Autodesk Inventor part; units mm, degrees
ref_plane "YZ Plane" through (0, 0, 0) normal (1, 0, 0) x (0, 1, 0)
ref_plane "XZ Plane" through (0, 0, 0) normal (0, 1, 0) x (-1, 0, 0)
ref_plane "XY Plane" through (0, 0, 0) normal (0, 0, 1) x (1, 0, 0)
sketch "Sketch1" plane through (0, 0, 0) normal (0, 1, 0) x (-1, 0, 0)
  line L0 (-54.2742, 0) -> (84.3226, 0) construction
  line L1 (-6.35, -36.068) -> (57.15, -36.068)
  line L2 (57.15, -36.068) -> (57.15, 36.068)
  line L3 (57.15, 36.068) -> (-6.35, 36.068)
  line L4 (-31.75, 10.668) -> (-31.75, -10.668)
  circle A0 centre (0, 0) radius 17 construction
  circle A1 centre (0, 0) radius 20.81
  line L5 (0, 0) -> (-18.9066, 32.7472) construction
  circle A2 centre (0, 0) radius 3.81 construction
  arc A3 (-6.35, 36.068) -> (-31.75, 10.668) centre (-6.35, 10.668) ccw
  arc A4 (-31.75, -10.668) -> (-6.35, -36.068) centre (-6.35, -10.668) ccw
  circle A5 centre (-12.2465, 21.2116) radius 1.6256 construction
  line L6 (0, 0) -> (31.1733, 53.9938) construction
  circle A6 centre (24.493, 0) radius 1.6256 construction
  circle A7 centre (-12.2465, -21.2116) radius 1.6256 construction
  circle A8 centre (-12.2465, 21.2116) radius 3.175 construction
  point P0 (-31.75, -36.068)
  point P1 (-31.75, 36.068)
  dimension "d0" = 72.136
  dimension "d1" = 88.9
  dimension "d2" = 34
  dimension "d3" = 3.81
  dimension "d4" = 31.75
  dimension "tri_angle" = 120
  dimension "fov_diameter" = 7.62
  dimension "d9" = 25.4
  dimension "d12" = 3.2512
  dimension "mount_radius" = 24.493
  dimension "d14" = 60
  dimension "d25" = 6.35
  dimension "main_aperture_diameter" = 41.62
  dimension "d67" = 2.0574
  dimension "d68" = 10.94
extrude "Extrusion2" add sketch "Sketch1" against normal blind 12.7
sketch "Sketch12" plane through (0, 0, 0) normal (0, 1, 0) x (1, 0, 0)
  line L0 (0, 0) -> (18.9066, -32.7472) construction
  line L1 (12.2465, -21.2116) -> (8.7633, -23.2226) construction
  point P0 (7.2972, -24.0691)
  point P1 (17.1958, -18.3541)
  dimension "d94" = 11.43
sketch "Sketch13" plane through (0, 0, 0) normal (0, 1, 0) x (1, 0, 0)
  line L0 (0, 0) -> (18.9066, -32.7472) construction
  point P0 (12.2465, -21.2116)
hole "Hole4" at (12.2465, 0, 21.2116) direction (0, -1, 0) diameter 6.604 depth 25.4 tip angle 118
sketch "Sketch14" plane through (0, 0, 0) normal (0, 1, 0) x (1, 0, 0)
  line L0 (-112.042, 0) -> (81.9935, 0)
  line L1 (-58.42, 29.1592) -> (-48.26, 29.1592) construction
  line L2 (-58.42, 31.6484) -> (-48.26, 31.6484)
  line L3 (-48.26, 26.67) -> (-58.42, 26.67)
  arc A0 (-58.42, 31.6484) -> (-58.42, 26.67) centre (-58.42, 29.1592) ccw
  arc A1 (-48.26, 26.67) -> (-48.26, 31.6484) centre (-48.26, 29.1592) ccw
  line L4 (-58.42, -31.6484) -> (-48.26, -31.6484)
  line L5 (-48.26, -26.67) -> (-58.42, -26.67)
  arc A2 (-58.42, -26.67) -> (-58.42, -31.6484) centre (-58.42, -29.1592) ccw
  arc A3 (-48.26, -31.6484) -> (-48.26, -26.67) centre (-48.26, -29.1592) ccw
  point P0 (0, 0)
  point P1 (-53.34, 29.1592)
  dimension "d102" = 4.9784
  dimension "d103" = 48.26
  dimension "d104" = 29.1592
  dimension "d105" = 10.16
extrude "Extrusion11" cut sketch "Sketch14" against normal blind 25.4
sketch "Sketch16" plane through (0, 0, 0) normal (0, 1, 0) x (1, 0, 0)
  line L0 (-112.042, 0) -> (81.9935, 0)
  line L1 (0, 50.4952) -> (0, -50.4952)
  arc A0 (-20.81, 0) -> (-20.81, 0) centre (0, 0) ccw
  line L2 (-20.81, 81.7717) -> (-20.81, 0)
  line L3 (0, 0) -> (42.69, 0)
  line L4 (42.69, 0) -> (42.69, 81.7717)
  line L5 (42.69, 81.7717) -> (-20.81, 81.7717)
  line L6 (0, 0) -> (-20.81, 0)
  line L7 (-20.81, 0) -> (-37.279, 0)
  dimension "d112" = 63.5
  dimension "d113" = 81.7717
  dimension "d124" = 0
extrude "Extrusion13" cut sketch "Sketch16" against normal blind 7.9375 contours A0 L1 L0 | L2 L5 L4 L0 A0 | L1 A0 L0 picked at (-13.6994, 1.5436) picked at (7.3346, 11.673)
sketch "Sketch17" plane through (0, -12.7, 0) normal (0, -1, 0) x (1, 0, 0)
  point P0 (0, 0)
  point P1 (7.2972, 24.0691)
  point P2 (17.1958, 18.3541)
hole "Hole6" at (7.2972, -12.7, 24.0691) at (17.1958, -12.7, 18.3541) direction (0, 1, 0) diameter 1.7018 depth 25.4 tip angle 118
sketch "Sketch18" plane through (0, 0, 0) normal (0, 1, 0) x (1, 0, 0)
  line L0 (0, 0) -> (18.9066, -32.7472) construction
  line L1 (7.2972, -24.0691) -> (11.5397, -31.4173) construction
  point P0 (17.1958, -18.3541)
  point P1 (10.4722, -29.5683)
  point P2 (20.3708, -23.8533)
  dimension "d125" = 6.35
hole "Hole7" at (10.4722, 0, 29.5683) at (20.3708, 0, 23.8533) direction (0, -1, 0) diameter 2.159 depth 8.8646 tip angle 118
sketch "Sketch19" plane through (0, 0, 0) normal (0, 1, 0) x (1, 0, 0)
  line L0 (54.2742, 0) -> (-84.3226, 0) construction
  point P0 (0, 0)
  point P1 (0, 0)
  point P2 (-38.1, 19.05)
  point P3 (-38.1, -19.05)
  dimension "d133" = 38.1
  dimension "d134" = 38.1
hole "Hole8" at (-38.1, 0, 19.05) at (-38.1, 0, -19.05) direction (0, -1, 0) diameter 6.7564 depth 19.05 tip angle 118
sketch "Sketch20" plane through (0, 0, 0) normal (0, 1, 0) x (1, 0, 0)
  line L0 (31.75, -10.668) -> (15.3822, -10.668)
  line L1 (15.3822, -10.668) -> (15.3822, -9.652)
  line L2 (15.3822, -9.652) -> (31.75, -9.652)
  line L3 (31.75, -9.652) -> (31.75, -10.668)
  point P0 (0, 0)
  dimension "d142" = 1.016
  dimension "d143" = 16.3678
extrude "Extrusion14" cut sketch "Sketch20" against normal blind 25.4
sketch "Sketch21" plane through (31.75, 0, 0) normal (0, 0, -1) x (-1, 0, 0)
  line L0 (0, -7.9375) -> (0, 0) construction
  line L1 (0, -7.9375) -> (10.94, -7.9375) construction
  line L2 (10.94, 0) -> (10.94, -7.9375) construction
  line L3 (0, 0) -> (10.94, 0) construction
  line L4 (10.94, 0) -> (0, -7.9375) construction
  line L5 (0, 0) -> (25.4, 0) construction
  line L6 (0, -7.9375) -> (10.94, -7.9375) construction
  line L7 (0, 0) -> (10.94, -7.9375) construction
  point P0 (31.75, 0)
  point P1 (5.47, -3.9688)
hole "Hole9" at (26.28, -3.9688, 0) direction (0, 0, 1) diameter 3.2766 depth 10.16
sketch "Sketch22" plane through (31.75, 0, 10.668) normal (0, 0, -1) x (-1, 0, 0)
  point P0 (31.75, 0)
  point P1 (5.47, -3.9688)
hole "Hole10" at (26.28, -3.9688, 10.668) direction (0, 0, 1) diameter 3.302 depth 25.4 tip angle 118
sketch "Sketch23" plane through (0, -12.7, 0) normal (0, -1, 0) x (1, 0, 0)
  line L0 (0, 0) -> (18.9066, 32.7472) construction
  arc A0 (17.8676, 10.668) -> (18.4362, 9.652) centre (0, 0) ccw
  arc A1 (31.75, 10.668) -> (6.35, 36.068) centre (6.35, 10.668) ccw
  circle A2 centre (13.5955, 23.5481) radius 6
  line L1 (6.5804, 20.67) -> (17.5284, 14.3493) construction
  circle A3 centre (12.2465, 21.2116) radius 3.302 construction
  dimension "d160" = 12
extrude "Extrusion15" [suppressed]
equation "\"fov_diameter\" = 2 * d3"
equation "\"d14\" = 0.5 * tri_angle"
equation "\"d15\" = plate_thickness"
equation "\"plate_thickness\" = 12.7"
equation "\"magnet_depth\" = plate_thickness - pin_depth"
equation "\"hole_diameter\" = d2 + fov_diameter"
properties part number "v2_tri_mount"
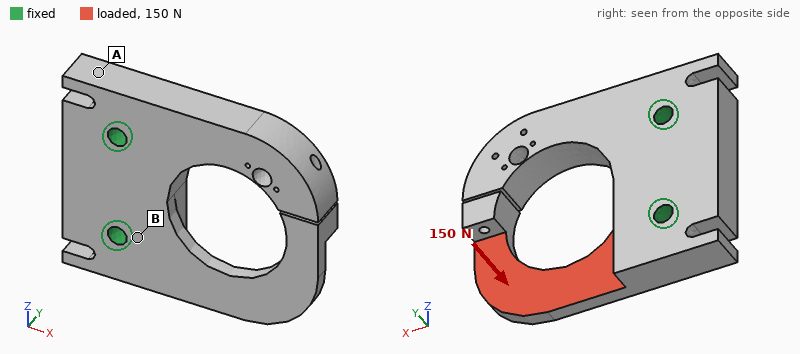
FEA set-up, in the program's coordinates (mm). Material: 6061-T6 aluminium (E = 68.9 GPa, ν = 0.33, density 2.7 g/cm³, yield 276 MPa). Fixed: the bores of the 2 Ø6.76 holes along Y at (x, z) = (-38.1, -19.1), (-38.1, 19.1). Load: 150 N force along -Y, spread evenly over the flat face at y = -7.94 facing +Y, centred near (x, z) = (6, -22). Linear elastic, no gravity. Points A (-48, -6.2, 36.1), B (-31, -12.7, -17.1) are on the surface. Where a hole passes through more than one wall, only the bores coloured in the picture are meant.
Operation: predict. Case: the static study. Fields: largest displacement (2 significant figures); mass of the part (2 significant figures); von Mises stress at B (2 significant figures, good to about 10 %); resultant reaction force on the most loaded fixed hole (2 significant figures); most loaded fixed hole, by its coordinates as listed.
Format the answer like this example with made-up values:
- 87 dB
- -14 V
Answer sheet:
- 0.37 mm
- 130 g
- 8.5 MPa
- 160 N
- (-38.1, -19.1)
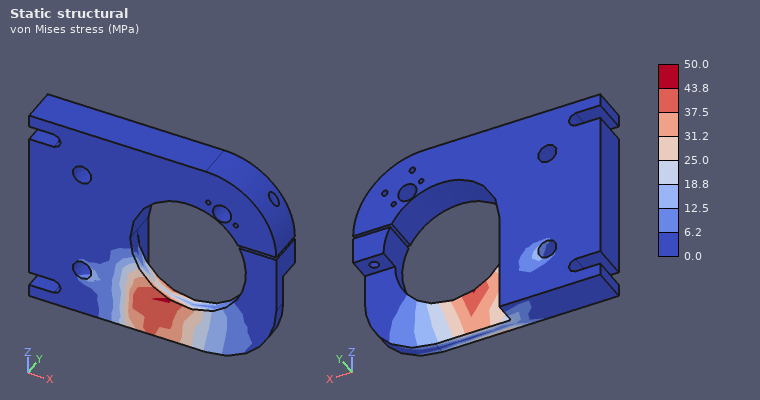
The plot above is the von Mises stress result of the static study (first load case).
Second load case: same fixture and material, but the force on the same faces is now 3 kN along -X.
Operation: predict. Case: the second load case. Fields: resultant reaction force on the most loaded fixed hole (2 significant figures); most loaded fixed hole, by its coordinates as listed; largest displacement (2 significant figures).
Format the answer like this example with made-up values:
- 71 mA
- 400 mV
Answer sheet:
- 3.1 kN
- (-38.1, -19.1)
- 0.74 mm
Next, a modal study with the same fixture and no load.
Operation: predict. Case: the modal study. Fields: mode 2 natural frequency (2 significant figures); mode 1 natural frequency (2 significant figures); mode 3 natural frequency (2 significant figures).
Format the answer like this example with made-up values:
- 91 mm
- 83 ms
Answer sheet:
- 2100 Hz
- 760 Hz
- 2600 Hz
